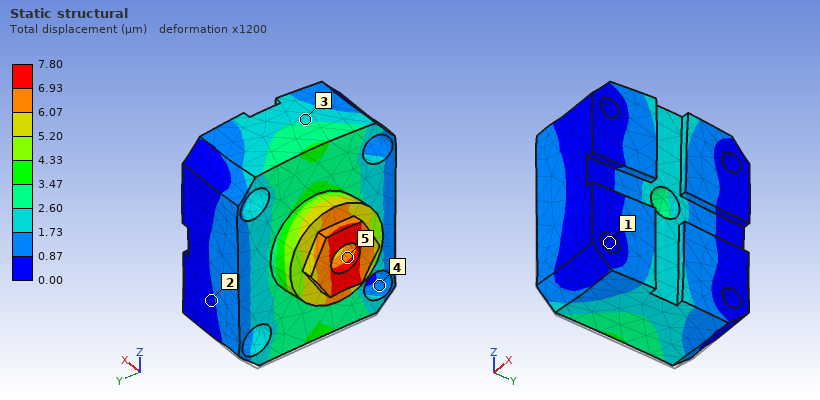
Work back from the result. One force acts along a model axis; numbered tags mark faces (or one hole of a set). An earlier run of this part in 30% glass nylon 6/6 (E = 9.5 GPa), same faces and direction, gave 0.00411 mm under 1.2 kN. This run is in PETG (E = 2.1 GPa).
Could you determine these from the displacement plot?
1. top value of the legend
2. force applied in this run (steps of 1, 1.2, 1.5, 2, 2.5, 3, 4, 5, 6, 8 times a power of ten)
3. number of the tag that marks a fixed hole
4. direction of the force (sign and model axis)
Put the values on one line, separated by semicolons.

7.80 µm; 500 N; 1; +Z
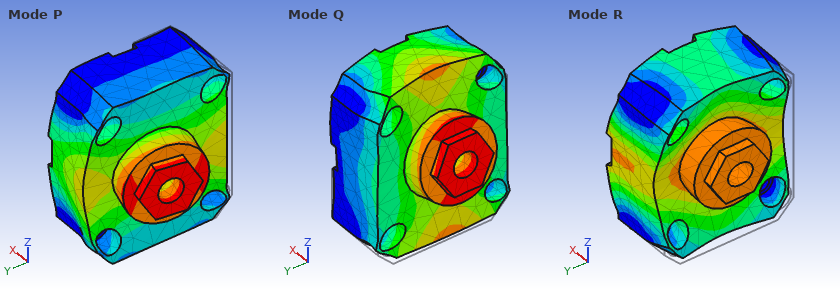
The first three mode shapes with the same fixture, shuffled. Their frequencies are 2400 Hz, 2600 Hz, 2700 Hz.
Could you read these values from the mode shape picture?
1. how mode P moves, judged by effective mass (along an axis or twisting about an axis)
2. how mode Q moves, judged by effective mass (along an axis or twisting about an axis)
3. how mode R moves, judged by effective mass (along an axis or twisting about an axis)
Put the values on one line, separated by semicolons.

along Y; along Z; along X
